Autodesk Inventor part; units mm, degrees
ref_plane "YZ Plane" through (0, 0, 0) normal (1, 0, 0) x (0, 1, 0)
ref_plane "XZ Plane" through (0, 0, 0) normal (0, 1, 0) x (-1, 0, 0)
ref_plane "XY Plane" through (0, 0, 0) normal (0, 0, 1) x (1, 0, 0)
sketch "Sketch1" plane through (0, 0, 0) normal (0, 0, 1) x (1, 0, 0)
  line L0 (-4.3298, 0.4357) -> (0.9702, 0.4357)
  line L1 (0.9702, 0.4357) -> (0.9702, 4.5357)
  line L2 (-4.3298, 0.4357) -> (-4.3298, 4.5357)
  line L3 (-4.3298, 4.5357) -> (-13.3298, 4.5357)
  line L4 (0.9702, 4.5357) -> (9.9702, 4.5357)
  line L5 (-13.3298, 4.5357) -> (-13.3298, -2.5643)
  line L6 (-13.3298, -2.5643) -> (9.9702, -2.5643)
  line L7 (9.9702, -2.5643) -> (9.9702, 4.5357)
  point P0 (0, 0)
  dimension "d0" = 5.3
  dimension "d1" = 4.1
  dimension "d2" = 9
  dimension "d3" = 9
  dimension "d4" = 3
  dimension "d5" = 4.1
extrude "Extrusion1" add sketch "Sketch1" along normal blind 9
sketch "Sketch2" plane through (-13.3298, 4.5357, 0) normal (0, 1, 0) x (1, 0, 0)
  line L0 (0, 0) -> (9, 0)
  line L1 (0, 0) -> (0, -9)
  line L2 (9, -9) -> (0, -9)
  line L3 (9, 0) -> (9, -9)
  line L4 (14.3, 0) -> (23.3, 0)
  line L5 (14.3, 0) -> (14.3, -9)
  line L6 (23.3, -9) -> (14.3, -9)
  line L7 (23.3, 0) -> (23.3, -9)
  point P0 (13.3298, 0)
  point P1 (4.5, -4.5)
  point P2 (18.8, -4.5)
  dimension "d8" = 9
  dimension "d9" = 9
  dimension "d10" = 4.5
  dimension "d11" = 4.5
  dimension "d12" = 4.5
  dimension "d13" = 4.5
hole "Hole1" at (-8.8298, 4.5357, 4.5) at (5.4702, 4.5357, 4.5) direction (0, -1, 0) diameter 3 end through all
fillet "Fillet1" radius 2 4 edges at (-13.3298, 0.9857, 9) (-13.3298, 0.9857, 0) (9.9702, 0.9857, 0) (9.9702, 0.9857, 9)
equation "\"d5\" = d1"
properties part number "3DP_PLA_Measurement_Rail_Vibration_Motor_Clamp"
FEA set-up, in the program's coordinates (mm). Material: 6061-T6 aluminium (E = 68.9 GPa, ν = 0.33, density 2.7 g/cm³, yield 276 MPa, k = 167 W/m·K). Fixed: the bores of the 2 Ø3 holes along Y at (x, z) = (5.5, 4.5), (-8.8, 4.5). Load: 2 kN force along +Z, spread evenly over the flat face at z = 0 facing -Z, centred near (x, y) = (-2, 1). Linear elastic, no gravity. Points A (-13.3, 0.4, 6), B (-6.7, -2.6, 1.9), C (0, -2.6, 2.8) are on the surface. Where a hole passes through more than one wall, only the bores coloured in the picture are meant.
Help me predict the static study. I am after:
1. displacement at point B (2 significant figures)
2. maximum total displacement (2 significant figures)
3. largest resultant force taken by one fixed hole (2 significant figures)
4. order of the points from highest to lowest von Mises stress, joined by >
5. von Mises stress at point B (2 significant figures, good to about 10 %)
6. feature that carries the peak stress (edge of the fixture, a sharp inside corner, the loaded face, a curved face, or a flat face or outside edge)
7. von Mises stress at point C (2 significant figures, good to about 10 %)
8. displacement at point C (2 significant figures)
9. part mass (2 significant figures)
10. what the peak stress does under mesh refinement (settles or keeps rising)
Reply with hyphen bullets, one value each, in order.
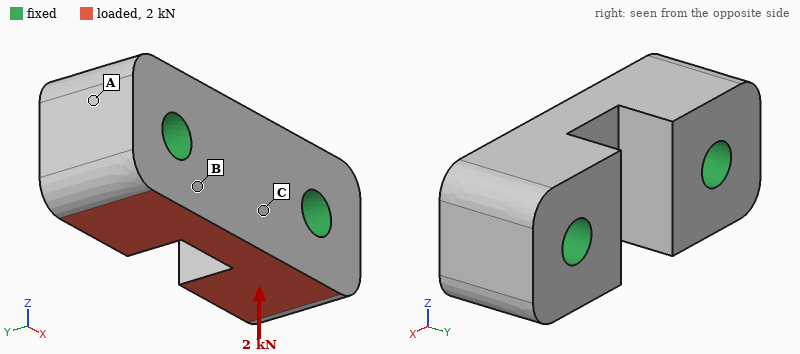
- 1.3 µm
- 3.3 µm
- 1.0 kN
- B > C > A
- 24 MPa
- edge of the fixture
- 14 MPa
- 2.5 µm
- 3.2 g
- keeps rising
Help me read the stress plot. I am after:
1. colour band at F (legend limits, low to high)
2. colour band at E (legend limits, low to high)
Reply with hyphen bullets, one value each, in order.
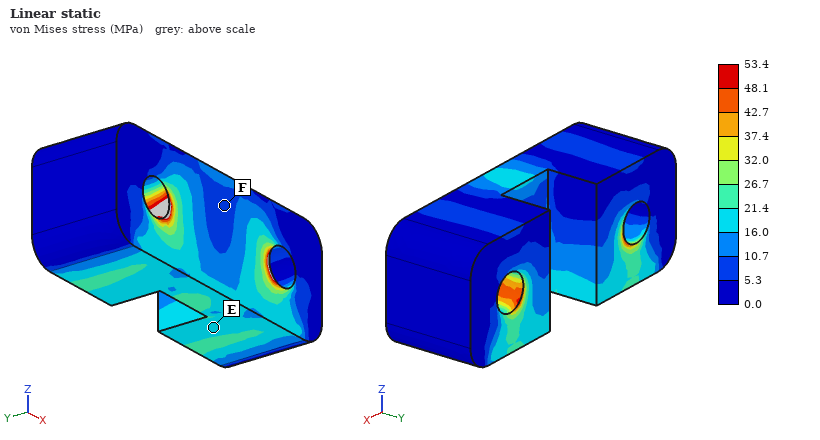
- 5.3 to 10.7 MPa
- 16.0 to 21.4 MPa
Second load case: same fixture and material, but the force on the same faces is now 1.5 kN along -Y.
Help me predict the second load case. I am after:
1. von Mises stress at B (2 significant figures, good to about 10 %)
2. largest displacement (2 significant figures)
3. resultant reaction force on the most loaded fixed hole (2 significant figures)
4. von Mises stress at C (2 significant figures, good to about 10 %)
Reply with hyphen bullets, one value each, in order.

- 35 MPa
- 8.2 µm
- 750 N
- 27 MPa
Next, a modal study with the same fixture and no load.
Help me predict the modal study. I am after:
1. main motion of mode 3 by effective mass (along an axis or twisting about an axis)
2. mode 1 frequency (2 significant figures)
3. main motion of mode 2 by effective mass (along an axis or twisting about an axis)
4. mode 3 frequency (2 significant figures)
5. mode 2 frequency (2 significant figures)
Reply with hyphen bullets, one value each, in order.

- twisting about Y
- 90 kHz
- along Y
- 110 kHz
- 100 kHz
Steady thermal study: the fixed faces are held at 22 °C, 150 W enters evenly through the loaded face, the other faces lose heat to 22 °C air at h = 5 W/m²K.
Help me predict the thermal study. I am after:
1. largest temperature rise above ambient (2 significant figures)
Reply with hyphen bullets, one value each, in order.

- 42 K
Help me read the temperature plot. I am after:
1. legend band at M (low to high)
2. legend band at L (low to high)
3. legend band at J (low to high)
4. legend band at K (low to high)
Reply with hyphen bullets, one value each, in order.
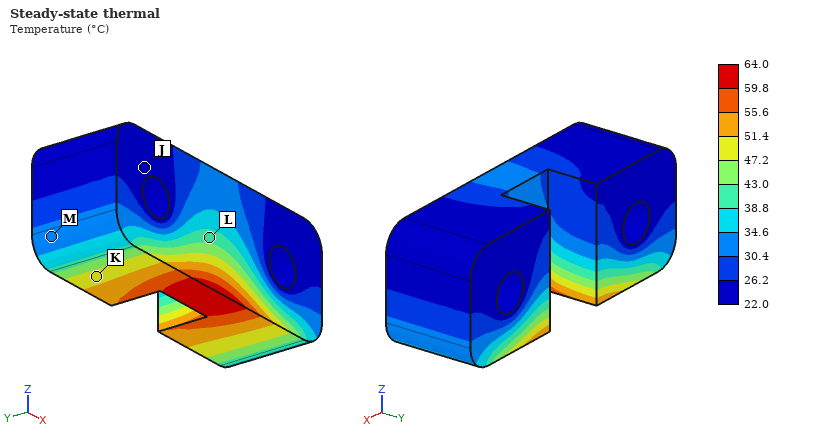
- 30.4 to 34.6 °C
- 38.8 to 43.0 °C
- 22.0 to 26.2 °C
- 47.2 to 51.4 °C
